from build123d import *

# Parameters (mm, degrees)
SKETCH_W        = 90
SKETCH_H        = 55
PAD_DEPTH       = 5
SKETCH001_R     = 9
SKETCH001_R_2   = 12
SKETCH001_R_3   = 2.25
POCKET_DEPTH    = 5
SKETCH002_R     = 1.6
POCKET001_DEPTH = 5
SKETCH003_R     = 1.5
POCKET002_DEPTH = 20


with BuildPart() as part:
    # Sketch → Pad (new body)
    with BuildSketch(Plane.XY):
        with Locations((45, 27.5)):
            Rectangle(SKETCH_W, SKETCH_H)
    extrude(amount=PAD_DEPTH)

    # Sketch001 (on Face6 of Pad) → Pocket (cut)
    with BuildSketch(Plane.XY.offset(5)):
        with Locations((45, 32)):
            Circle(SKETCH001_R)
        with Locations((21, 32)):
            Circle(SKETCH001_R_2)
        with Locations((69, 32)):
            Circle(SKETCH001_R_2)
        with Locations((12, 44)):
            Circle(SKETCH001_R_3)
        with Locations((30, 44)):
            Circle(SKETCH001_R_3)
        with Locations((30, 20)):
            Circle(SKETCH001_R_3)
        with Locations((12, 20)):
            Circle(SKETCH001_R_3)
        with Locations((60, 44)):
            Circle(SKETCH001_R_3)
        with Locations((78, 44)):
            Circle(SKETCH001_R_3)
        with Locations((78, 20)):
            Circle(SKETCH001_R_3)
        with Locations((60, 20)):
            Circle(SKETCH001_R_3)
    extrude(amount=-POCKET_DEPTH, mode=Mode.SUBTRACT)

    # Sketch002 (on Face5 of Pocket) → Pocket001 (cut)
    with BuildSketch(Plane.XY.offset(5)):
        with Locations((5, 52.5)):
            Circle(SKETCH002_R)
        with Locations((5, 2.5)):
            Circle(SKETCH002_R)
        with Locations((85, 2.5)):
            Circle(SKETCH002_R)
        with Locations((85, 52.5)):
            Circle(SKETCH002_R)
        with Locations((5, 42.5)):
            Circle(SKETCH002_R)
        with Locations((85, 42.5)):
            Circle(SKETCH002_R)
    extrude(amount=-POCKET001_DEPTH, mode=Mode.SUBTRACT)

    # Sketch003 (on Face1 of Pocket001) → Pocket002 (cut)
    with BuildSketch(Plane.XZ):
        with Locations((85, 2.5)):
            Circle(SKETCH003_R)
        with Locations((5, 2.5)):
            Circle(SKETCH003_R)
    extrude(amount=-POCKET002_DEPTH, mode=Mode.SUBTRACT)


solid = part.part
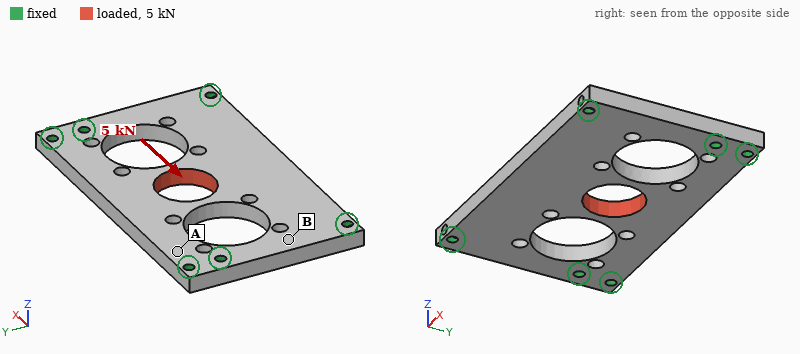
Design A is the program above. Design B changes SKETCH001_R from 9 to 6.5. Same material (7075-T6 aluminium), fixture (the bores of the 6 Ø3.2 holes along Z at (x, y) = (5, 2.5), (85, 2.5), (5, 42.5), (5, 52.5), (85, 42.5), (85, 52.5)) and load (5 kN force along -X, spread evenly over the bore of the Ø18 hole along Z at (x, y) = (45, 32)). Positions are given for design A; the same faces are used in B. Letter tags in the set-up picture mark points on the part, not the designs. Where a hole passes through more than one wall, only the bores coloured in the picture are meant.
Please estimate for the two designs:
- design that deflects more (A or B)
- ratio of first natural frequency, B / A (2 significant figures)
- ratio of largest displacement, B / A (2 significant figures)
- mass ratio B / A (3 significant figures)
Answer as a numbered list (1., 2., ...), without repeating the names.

1. A
2. 0.98
3. 0.87
4. 1.03
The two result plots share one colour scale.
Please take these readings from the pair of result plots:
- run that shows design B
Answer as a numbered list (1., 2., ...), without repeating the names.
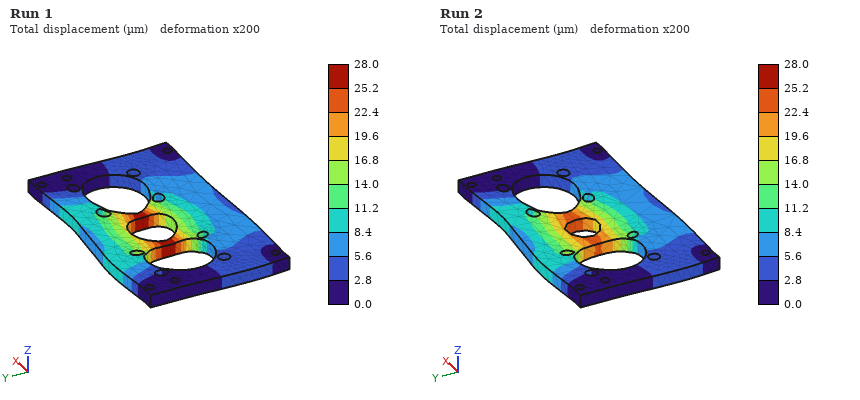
1. Run 2
